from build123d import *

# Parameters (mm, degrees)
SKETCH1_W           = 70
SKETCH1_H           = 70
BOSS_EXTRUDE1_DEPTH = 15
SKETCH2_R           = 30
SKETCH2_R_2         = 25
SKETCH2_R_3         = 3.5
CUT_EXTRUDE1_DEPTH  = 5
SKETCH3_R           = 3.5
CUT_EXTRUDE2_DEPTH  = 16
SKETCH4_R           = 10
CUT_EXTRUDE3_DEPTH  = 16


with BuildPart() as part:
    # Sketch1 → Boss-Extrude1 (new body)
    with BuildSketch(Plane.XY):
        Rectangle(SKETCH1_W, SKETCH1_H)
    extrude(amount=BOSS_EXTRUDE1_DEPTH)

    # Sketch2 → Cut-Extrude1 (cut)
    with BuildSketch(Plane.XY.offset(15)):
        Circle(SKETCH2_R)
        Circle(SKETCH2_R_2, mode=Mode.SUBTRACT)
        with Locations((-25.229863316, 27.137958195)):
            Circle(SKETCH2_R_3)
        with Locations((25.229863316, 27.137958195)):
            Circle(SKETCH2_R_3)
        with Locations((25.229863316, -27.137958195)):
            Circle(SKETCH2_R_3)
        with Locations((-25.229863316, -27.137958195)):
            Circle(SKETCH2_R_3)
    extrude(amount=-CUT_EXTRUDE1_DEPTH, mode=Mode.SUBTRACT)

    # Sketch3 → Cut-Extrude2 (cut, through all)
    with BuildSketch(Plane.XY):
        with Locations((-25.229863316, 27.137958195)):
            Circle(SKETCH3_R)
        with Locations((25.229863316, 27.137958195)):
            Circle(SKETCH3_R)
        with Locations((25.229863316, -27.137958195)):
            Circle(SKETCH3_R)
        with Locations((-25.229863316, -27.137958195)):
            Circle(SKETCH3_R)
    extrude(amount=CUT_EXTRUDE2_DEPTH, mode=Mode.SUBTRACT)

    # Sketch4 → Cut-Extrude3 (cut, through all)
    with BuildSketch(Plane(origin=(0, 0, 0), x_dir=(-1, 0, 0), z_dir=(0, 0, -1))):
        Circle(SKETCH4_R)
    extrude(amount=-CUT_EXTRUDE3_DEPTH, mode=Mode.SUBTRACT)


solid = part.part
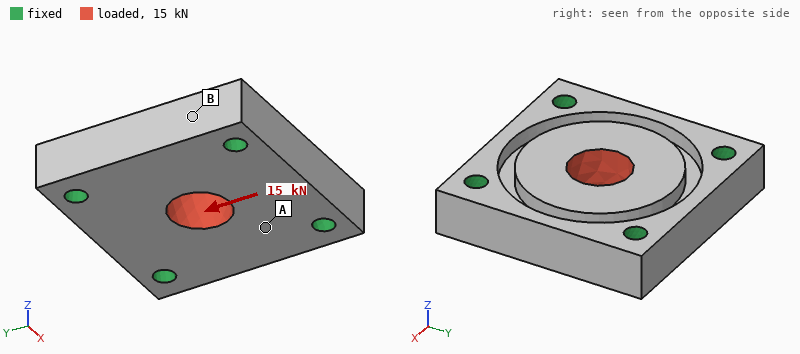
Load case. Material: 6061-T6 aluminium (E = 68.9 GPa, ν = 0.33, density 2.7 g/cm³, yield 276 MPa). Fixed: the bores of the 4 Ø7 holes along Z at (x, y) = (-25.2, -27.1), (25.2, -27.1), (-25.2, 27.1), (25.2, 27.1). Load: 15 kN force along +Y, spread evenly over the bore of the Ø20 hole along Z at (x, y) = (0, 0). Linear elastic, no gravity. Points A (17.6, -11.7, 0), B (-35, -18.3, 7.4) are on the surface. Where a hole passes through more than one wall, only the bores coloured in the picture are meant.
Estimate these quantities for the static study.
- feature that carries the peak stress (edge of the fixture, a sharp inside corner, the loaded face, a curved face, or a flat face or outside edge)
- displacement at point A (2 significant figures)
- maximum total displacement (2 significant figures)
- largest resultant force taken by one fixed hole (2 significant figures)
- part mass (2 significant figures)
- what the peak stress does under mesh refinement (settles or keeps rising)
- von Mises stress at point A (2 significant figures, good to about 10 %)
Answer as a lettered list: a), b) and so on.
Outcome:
a) edge of the fixture
b) 4.1 µm
c) 11 µm
d) 4.1 kN
e) 170 g
f) keeps rising
g) 15 MPa
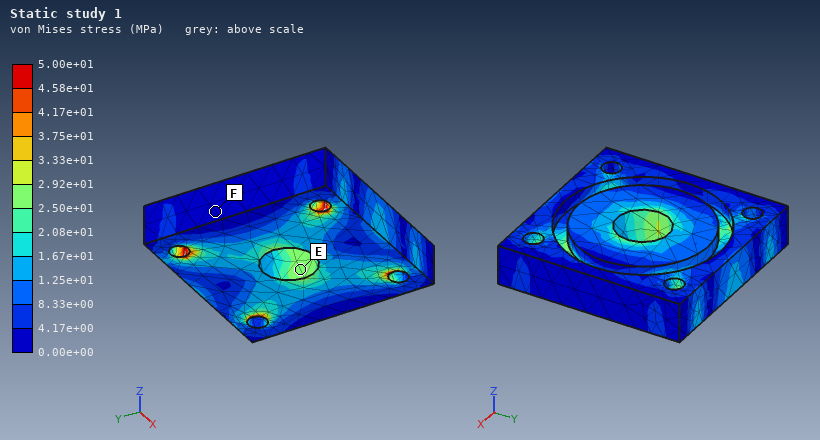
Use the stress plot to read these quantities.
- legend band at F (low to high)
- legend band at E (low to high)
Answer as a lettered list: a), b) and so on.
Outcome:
a) 0.00e+00 to 4.17e+00 MPa
b) 2.50e+01 to 2.92e+01 MPa
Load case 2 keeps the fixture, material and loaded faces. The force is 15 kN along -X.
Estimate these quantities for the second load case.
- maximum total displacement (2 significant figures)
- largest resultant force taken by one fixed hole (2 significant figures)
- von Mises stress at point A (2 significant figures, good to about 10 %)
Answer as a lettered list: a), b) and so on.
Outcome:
a) 12 µm
b) 4.0 kN
c) 14 MPa
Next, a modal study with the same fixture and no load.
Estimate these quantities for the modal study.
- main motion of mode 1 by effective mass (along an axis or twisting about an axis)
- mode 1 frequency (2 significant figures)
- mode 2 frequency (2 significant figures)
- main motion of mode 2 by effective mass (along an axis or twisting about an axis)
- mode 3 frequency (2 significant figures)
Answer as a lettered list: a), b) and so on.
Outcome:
a) along Z
b) 15 kHz
c) 20 kHz
d) twisting about Y
e) 22 kHz
